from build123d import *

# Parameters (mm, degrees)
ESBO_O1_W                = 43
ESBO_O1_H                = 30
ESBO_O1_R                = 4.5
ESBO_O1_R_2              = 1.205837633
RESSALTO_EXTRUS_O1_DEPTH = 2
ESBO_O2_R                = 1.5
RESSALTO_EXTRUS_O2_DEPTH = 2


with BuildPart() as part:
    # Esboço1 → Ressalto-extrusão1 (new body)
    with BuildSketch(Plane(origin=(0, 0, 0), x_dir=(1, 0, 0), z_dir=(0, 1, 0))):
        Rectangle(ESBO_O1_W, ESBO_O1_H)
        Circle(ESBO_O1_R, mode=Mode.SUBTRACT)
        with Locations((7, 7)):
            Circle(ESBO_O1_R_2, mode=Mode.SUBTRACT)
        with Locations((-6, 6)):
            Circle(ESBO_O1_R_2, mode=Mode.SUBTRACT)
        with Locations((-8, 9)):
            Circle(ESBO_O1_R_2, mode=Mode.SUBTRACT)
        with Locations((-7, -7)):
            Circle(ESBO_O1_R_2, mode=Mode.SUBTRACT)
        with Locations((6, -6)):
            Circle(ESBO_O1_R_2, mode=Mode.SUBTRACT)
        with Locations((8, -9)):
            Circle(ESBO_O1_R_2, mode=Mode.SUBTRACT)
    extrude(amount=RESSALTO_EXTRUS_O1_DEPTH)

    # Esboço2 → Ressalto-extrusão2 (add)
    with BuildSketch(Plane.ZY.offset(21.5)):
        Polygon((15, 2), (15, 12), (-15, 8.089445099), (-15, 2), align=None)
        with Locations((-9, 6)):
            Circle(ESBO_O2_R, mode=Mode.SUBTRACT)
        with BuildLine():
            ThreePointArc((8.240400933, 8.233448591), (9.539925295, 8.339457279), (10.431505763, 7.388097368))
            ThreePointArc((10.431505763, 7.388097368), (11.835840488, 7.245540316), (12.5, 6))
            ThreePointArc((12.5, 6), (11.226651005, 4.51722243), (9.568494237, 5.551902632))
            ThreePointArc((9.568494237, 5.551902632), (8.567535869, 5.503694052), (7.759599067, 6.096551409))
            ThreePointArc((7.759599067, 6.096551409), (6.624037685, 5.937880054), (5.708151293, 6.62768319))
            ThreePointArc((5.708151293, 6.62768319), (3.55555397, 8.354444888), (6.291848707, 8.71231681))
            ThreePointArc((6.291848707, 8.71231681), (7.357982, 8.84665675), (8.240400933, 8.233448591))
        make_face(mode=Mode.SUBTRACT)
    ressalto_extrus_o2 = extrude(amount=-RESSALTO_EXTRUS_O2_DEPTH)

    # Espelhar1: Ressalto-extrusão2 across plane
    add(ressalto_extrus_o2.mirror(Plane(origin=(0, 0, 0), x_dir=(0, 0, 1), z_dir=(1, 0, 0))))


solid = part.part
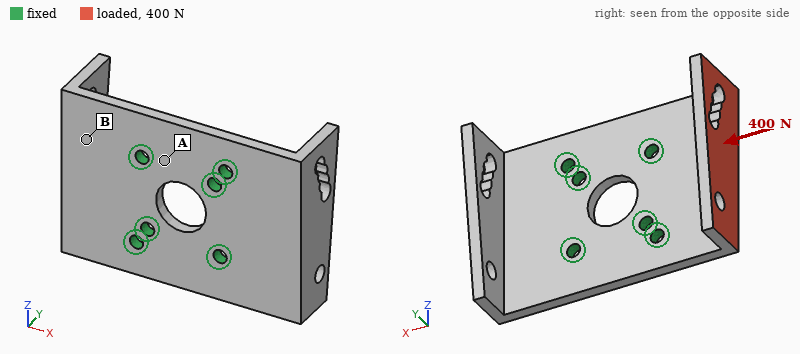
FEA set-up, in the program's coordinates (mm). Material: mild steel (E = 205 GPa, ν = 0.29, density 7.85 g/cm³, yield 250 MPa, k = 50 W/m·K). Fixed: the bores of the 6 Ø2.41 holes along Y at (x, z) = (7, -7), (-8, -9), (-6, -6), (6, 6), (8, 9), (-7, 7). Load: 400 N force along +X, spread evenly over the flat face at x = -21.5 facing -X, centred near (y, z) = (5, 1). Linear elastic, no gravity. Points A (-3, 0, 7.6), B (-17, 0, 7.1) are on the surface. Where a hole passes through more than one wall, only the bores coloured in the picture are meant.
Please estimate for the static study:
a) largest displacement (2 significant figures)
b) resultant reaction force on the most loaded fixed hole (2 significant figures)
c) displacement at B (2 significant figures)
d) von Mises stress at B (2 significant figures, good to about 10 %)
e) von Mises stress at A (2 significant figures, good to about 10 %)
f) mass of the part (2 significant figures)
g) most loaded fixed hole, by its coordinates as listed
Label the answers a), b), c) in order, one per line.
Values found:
a) 85 µm
b) 180 N
c) 19 µm
d) 61 MPa
e) 15 MPa
f) 25 g
g) (-7, 7)
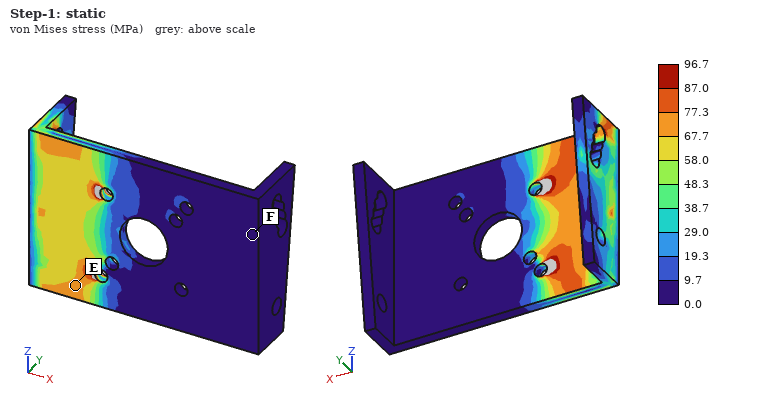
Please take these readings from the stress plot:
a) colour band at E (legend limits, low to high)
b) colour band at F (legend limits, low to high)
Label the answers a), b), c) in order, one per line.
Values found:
a) 67.7 to 77.3 MPa
b) 0.0 to 9.7 MPa
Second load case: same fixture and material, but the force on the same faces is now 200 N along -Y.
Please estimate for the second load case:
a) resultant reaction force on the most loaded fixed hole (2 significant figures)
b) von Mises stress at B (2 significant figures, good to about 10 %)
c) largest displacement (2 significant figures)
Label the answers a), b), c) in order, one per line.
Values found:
a) 140 N
b) 37 MPa
c) 77 µm
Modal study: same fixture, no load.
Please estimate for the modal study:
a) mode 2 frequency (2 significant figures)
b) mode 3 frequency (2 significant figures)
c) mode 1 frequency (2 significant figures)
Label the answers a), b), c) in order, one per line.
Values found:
a) 4500 Hz
b) 7200 Hz
c) 4500 Hz
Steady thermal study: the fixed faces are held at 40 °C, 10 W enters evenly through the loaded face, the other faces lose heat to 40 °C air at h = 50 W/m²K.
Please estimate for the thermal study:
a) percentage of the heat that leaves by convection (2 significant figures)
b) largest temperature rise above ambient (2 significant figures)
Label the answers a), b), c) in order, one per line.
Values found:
a) 19 %
b) 62 K
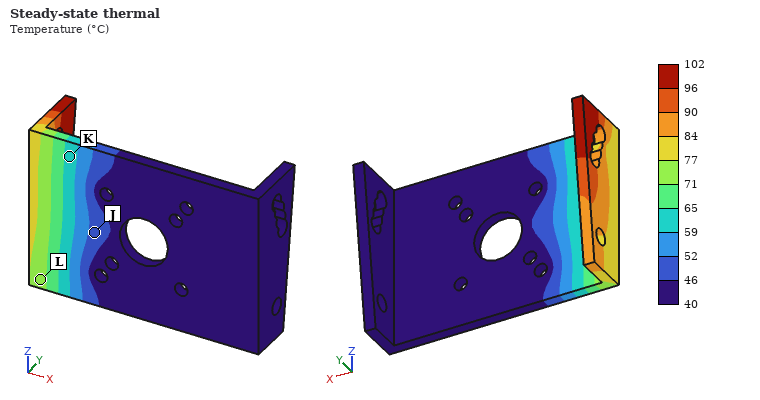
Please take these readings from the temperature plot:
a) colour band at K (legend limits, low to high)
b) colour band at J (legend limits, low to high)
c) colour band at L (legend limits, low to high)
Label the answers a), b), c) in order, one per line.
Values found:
a) 59 to 65 °C
b) 46 to 52 °C
c) 71 to 77 °C
